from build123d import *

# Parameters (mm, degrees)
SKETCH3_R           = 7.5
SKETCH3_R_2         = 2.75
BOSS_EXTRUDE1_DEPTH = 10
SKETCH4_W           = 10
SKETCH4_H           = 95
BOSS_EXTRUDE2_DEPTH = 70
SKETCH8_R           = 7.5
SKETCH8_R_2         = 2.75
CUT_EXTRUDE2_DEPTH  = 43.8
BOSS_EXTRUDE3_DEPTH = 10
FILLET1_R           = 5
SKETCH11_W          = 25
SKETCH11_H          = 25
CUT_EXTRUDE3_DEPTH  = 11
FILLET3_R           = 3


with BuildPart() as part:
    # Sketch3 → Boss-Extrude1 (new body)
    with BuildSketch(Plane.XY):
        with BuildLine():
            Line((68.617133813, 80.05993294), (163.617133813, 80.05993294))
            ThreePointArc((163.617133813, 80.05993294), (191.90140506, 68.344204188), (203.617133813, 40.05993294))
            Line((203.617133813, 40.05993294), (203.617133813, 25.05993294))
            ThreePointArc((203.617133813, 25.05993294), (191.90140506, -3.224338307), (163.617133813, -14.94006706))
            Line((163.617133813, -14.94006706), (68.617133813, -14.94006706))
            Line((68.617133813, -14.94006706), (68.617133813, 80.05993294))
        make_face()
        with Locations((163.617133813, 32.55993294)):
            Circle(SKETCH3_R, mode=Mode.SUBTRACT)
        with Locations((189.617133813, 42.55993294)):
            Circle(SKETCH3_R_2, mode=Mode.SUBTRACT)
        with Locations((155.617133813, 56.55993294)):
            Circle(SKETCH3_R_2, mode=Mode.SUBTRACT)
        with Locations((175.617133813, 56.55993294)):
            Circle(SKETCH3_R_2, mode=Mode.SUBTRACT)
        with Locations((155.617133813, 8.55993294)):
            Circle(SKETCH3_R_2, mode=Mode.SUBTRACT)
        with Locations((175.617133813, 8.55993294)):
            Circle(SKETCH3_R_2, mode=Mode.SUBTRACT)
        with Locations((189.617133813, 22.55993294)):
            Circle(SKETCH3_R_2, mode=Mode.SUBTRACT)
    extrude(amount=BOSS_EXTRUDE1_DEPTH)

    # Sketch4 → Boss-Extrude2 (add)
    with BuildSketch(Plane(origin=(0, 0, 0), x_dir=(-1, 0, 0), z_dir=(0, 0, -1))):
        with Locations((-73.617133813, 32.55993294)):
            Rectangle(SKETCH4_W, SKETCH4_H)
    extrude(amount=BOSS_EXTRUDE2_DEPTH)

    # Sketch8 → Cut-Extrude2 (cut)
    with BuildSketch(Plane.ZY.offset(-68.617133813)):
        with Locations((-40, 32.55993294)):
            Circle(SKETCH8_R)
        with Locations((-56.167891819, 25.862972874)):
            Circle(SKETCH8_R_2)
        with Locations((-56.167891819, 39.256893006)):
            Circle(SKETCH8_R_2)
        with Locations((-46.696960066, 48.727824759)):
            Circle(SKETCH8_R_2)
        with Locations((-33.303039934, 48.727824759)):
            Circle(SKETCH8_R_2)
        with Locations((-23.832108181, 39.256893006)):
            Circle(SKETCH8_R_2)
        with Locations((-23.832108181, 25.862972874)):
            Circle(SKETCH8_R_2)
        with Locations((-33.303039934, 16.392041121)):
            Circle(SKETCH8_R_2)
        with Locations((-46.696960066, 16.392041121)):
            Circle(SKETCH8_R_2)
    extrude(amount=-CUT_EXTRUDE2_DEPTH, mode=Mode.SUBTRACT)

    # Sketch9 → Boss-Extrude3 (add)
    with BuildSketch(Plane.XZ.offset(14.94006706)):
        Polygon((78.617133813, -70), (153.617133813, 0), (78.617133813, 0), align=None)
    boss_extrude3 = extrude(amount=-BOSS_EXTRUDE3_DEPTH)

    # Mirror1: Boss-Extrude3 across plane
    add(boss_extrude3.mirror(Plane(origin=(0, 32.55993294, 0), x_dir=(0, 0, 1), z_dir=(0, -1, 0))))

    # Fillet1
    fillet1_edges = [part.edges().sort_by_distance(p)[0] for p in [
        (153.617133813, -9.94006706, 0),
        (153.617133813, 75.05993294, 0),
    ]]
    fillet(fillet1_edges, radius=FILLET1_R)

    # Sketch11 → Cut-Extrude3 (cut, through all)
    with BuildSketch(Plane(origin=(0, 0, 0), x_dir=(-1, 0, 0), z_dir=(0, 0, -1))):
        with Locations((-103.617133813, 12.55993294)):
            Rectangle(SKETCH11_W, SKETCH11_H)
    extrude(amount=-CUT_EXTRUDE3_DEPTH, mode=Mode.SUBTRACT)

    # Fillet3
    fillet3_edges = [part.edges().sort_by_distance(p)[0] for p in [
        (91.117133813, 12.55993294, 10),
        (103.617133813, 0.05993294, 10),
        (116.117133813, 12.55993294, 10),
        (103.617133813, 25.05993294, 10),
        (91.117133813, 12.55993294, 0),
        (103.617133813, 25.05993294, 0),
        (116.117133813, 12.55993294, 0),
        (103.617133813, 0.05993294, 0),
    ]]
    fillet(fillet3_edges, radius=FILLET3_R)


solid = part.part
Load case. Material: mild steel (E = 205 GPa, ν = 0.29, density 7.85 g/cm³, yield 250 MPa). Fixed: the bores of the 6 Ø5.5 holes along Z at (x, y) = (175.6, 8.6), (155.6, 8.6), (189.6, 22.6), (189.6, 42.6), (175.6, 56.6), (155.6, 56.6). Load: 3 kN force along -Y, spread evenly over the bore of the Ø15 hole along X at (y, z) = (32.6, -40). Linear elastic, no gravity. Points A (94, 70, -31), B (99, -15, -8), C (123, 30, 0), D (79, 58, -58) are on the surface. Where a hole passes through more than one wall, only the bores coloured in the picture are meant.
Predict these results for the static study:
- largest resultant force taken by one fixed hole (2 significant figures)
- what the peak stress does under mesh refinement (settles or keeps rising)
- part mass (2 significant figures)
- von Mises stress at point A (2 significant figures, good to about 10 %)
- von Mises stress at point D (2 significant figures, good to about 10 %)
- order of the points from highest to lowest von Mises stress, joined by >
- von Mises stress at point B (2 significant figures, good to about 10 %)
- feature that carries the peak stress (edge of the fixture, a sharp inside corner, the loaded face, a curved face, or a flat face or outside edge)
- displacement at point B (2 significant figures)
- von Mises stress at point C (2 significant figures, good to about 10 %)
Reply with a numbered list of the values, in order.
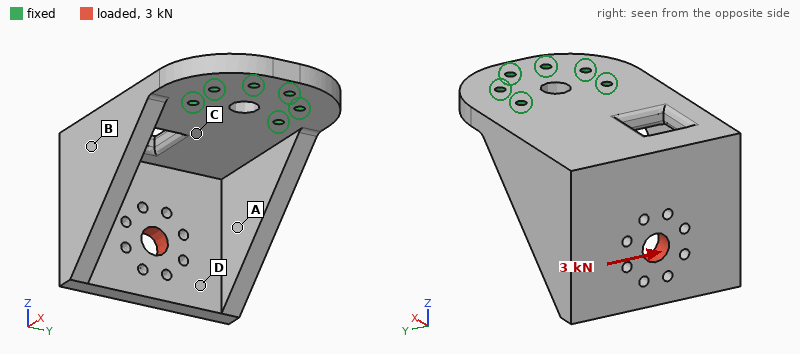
1. 4.2 kN
2. keeps rising
3. 1.8 kg
4. 18 MPa
5. 26 MPa
6. C > D > A > B
7. 12 MPa
8. edge of the fixture
9. 0.057 mm
10. 32 MPa
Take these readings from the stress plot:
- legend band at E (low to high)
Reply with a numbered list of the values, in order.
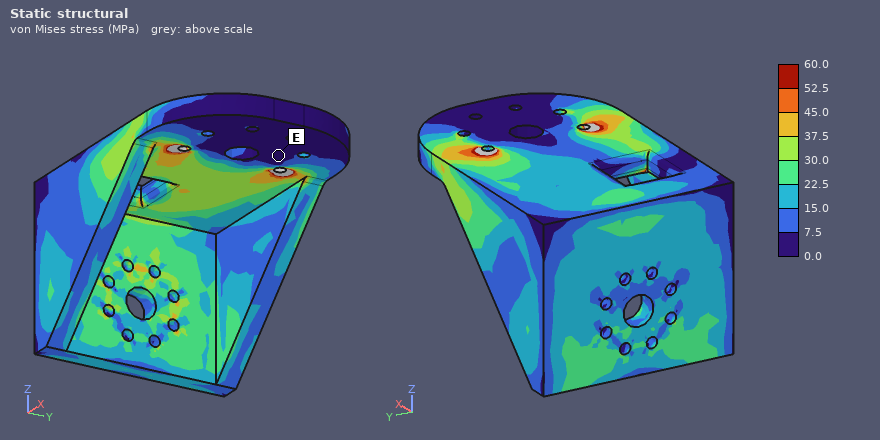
1. 0.0 to 7.5 MPa
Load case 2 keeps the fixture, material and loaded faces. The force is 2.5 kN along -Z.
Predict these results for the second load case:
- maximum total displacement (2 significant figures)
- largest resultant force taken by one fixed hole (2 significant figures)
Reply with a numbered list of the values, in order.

1. 0.27 mm
2. 3.6 kN
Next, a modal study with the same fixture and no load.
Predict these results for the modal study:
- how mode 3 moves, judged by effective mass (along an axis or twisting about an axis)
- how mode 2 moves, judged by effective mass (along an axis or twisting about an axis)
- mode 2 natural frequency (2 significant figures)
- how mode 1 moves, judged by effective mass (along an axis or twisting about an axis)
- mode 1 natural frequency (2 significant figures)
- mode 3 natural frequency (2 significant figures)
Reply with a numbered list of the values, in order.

1. along Y
2. along Y
3. 940 Hz
4. along Z
5. 560 Hz
6. 2900 Hz
